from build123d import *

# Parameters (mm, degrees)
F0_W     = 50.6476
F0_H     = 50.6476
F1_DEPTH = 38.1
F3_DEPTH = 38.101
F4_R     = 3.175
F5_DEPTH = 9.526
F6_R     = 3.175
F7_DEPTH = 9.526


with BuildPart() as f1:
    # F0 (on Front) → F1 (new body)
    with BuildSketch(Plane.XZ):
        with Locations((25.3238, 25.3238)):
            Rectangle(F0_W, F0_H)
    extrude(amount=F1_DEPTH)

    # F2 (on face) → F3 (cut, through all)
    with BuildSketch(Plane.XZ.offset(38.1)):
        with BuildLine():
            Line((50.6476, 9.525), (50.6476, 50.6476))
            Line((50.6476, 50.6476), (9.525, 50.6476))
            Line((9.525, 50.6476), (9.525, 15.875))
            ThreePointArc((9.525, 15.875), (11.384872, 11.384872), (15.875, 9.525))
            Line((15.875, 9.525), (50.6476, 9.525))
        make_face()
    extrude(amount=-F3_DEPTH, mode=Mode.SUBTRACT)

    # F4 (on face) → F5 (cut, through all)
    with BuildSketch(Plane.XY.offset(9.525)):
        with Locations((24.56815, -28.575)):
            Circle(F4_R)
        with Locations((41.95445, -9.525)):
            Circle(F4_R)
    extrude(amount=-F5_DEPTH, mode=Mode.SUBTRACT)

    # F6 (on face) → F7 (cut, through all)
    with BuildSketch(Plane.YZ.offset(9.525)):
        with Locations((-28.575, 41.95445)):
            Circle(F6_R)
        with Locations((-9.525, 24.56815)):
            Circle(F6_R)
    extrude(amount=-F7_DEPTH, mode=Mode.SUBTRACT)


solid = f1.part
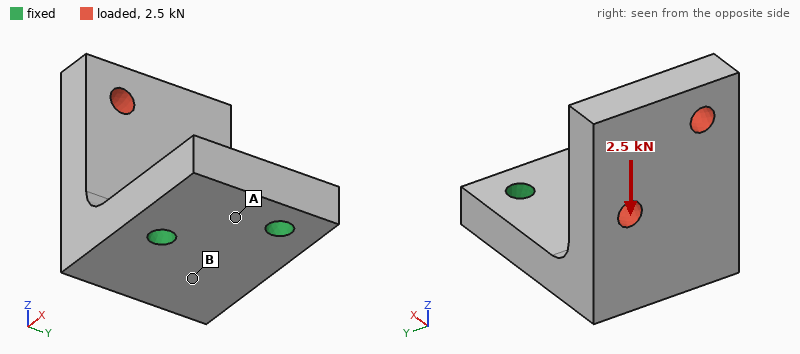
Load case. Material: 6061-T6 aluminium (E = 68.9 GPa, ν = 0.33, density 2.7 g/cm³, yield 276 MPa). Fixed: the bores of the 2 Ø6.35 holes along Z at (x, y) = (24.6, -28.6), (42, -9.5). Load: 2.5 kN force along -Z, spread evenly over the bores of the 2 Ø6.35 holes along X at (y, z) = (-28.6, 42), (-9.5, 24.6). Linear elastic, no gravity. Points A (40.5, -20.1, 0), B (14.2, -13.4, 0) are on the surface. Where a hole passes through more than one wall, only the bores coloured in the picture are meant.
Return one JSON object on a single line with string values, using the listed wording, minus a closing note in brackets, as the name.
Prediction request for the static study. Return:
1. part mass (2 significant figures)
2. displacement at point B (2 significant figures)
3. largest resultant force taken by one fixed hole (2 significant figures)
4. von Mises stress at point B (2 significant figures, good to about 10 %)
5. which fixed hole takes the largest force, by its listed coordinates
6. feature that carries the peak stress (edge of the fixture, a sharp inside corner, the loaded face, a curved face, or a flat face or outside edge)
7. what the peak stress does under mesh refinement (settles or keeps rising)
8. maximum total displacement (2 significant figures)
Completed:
{"part mass": "88 g", "displacement at point B": "0.039 mm", "largest resultant force taken by one fixed hole": "2.6 kN", "von Mises stress at point B": "28 MPa", "which fixed hole takes the largest force, by its listed coordinates": "(24.6, -28.6)", "feature that carries the peak stress": "edge of the fixture", "what the peak stress does under mesh refinement": "keeps rising", "maximum total displacement": "0.19 mm"}
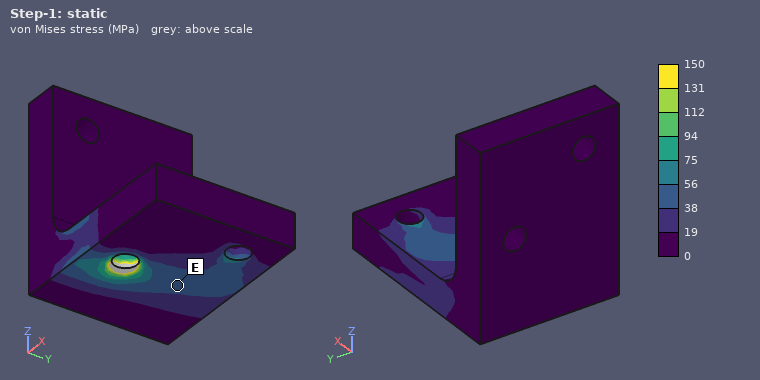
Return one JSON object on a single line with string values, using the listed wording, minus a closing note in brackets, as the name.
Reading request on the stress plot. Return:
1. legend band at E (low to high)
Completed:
{"legend band at E": "38 to 56 MPa"}
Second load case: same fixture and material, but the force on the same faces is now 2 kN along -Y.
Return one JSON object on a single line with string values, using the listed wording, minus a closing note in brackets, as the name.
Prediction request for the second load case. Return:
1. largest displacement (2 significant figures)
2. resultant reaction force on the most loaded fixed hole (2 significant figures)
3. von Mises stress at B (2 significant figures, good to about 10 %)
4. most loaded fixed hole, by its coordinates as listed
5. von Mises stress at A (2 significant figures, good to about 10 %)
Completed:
{"largest displacement": "0.19 mm", "resultant reaction force on the most loaded fixed hole": "2.8 kN", "von Mises stress at B": "32 MPa", "most loaded fixed hole, by its coordinates as listed": "(24.6, -28.6)", "von Mises stress at A": "12 MPa"}
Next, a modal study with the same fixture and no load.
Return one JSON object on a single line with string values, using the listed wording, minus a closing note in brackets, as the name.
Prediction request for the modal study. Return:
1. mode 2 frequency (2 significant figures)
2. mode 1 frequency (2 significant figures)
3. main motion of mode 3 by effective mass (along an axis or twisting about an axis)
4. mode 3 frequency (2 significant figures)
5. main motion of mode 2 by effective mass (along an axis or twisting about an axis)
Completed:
{"mode 2 frequency": "3400 Hz", "mode 1 frequency": "2300 Hz", "main motion of mode 3 by effective mass": "along Z", "mode 3 frequency": "7400 Hz", "main motion of mode 2 by effective mass": "along Y"}
